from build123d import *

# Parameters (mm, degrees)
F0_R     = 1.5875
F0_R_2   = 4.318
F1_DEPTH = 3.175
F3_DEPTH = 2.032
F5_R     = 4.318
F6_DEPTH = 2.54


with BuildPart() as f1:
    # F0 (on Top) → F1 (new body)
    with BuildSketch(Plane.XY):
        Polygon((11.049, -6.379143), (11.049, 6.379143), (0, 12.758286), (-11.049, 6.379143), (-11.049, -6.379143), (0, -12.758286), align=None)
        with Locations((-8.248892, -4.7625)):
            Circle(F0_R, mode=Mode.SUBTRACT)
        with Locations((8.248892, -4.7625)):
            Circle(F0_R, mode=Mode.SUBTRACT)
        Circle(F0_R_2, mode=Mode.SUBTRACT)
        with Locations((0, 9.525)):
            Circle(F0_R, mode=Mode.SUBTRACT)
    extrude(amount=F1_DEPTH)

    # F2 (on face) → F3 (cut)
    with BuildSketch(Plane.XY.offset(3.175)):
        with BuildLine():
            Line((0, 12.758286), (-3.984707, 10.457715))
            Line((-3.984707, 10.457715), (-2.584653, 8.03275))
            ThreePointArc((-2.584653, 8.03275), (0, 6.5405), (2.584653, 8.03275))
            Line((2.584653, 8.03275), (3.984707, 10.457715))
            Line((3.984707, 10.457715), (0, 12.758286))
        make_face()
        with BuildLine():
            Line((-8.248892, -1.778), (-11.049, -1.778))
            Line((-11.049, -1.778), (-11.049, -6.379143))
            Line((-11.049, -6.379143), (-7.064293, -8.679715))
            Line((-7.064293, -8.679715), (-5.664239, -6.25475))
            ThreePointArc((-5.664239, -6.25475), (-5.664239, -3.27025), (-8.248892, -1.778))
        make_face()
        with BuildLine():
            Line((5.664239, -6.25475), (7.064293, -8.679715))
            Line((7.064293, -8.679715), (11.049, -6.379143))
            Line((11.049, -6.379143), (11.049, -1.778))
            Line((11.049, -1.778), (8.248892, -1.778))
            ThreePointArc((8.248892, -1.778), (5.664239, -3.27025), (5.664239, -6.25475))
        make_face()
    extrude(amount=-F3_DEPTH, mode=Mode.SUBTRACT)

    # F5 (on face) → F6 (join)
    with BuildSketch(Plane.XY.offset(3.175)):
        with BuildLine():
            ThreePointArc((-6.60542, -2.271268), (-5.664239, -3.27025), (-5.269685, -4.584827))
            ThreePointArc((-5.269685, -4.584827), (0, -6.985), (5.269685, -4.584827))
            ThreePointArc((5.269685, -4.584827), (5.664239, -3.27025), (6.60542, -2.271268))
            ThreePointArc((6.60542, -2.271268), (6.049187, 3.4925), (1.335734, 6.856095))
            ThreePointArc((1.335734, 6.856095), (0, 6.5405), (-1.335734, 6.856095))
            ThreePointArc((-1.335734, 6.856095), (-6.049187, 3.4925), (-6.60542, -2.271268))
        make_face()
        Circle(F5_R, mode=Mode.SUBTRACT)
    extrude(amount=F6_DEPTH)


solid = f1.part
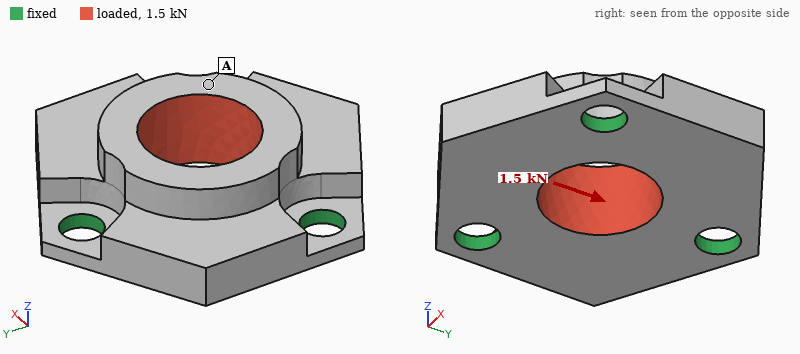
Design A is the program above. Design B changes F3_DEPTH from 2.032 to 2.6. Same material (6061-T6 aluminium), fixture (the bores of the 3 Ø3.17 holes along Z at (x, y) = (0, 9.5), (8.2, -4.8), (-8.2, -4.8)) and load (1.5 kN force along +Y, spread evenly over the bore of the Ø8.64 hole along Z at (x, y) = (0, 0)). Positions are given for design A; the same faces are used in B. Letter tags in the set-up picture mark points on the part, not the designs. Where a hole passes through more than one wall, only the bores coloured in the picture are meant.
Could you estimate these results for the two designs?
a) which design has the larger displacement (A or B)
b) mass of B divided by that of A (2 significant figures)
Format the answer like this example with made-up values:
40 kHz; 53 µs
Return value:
B; 0.97
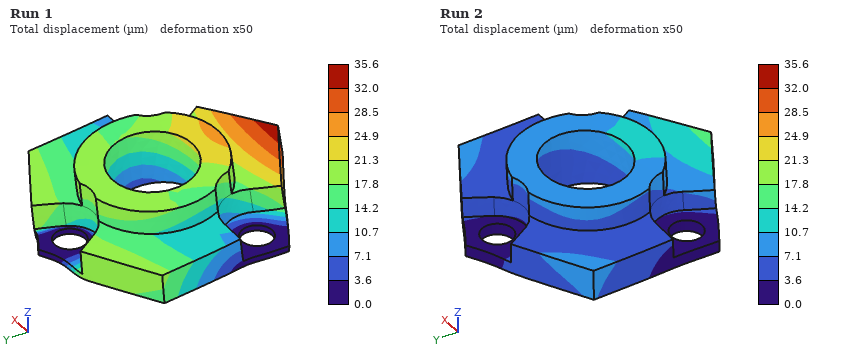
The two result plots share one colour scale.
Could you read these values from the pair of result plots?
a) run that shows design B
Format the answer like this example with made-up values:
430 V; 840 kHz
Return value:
Run 1
